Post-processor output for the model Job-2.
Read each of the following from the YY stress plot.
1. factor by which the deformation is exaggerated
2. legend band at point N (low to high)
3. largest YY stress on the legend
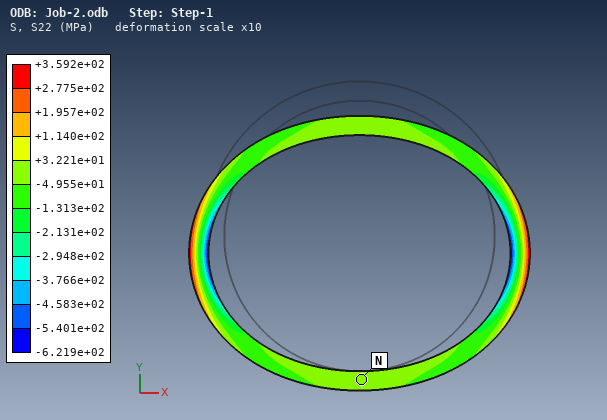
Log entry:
10
-4.955e+01 to +3.221e+01 MPa
+3.592e+02 MPa
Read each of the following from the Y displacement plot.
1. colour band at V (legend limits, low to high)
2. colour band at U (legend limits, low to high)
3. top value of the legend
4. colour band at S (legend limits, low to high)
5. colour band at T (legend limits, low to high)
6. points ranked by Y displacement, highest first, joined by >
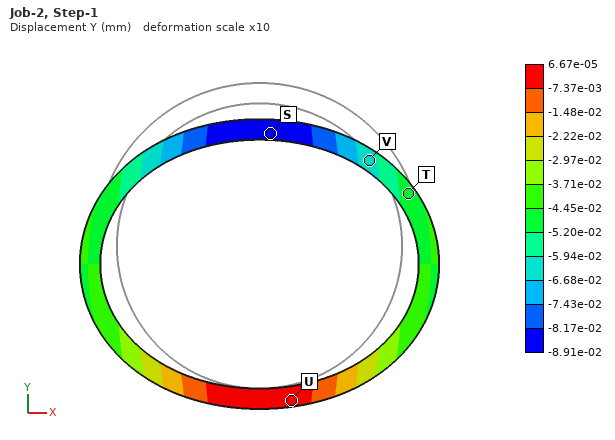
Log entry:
-6.68e-02 to -5.94e-02 mm
-7.37e-03 to 6.67e-05 mm
6.67e-05 mm
-8.91e-02 to -8.17e-02 mm
-5.20e-02 to -4.45e-02 mm
U > T > V > S
